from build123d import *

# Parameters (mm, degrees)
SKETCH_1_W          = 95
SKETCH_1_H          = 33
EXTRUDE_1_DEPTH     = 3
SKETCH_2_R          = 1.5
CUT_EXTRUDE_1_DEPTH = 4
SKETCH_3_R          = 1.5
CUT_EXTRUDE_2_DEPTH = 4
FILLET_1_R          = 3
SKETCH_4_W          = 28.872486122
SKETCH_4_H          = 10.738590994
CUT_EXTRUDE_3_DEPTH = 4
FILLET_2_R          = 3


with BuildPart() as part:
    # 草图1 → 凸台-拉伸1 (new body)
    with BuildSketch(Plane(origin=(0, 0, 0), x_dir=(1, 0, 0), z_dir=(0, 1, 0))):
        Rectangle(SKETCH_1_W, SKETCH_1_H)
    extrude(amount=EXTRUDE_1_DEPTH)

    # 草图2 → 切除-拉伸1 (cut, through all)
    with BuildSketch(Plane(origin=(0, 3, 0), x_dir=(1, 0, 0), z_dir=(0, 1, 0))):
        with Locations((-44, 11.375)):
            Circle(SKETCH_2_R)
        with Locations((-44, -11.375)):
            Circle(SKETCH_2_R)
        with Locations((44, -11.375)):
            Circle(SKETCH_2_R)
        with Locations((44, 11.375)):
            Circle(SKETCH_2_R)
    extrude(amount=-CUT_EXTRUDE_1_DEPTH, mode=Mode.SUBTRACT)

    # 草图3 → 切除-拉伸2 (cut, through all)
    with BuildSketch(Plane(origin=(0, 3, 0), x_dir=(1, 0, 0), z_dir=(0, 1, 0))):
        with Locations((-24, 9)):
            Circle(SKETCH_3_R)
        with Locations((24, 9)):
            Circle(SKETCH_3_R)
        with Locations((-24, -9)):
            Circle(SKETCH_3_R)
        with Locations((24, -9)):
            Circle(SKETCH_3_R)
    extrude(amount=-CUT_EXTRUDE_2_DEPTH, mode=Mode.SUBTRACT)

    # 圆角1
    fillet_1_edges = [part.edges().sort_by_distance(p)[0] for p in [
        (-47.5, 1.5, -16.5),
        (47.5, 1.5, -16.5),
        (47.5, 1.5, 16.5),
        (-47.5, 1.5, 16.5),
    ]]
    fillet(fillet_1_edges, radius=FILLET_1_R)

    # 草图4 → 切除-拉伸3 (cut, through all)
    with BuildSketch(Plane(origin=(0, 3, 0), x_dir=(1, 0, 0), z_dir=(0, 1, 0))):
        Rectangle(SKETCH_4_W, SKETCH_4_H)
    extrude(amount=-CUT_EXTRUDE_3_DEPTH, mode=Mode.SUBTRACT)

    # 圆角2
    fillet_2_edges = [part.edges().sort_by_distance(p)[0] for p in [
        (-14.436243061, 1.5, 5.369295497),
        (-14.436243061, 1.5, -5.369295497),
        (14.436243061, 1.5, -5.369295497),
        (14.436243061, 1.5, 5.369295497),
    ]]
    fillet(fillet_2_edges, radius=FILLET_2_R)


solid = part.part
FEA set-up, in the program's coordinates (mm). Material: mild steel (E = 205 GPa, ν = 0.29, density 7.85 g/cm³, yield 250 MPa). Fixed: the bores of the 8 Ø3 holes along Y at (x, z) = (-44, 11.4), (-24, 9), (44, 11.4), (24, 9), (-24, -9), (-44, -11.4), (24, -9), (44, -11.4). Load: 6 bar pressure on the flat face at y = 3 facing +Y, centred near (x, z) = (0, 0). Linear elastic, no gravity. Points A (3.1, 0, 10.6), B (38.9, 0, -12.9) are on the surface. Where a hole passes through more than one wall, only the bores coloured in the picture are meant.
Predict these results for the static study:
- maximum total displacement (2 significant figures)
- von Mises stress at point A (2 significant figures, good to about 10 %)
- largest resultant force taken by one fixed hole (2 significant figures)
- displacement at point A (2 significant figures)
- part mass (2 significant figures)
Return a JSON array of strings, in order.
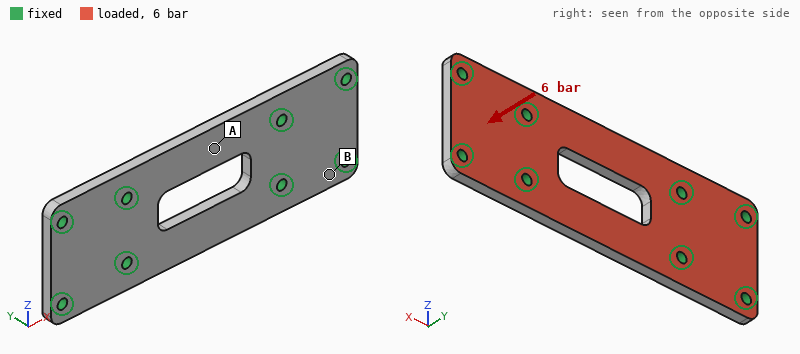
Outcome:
["17 µm", "31 MPa", "300 N", "15 µm", "65 g"]
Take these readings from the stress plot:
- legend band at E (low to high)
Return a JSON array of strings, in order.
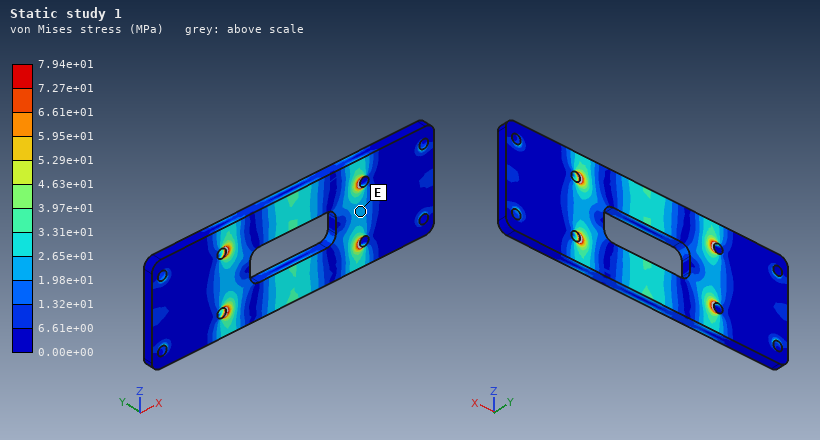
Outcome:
["1.98e+01 to 2.65e+01 MPa"]
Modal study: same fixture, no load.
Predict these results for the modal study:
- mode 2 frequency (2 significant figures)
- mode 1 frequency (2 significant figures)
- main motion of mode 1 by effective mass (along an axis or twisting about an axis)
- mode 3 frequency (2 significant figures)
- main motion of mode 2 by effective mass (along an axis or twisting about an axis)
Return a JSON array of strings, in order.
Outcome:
["7700 Hz", "7300 Hz", "along Y", "17 kHz", "twisting about X"]
